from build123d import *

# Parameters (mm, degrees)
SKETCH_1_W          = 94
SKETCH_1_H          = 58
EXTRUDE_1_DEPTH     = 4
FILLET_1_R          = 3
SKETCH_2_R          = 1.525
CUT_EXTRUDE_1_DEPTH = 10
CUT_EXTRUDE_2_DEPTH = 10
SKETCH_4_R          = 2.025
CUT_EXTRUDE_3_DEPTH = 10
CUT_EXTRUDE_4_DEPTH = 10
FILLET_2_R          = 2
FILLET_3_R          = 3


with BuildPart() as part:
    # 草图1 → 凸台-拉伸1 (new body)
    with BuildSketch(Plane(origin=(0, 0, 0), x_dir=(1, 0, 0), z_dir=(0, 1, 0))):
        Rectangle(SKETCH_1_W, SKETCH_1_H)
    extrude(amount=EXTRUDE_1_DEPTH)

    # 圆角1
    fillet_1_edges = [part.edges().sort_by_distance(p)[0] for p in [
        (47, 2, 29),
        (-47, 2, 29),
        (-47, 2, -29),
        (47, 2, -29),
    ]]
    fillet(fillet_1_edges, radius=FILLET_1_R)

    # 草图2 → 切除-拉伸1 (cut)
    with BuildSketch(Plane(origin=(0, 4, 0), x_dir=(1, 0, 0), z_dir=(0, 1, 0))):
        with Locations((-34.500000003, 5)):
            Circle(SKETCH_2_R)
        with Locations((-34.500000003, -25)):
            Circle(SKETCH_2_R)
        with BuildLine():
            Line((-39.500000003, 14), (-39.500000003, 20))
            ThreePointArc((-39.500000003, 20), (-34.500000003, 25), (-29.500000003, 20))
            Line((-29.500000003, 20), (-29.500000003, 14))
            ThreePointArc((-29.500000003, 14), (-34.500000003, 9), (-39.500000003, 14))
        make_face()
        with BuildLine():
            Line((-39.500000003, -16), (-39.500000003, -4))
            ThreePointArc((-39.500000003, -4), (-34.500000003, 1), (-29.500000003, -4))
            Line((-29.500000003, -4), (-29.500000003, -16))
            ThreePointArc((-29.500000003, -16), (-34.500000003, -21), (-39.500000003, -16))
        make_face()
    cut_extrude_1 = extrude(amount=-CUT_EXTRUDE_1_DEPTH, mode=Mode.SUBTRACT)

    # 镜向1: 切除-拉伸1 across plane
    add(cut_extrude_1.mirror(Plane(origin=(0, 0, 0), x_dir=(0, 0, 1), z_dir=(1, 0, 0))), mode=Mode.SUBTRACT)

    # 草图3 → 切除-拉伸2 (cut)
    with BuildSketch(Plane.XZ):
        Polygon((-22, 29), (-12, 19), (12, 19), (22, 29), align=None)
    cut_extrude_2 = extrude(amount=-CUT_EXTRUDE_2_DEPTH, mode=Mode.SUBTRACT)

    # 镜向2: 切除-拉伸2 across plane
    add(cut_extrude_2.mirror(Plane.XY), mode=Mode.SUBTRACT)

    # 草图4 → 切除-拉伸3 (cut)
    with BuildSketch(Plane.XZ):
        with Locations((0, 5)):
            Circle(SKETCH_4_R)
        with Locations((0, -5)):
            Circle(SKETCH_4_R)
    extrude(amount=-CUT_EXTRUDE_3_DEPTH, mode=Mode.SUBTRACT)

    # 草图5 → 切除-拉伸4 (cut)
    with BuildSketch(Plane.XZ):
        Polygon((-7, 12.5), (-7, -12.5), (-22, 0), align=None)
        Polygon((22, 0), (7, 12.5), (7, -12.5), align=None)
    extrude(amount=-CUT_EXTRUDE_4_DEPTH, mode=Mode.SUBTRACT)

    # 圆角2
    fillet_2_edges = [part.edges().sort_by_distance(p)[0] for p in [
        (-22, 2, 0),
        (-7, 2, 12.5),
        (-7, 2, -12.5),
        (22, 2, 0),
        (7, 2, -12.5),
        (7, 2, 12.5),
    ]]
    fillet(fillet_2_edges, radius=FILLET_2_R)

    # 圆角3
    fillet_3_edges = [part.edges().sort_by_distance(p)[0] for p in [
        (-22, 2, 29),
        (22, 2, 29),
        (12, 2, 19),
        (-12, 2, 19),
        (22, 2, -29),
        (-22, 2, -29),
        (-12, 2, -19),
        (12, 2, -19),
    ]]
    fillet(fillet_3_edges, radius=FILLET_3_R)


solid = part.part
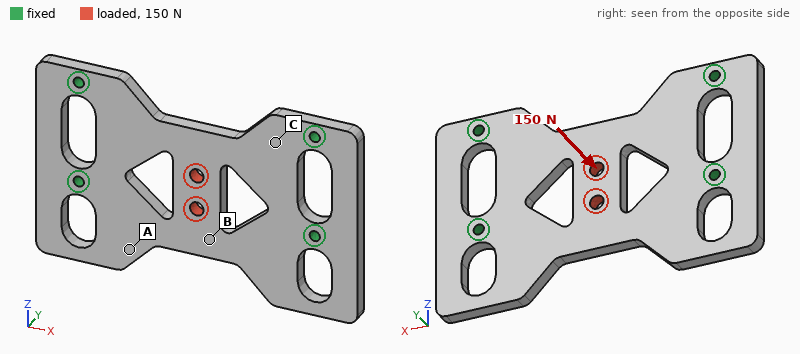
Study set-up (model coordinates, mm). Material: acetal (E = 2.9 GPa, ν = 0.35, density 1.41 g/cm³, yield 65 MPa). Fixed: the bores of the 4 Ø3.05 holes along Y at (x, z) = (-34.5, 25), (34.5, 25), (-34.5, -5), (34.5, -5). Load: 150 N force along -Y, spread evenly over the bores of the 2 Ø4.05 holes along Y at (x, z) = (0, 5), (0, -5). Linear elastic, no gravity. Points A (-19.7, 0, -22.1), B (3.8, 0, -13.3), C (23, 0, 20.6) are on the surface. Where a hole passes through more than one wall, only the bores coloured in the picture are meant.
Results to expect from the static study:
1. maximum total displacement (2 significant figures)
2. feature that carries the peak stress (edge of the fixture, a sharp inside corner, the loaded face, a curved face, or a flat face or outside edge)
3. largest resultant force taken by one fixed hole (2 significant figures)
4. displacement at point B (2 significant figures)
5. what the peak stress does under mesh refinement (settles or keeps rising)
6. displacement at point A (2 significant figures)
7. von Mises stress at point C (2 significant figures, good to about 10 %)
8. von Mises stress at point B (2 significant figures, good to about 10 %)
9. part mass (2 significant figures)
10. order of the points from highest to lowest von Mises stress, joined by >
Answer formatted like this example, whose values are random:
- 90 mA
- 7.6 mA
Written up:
- 0.88 mm
- edge of the fixture
- 58 N
- 0.78 mm
- keeps rising
- 0.39 mm
- 6.0 MPa
- 16 MPa
- 21 g
- B > C > A
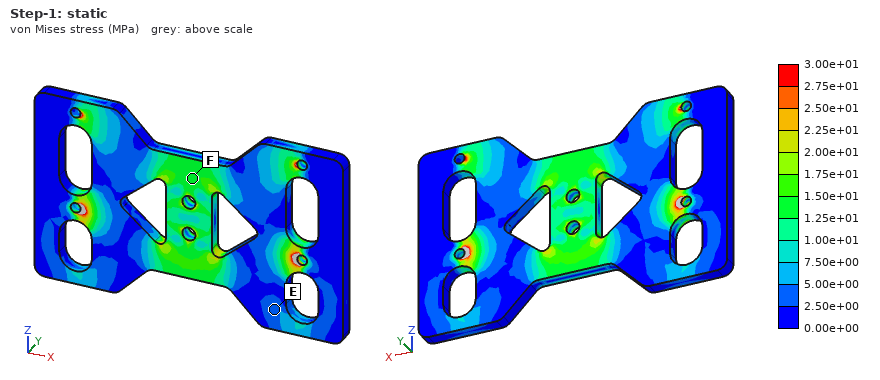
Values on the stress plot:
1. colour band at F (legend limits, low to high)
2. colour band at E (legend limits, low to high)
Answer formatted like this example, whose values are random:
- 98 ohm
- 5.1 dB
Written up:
- 1.25e+01 to 1.50e+01 MPa
- 2.50e+00 to 5.00e+00 MPa
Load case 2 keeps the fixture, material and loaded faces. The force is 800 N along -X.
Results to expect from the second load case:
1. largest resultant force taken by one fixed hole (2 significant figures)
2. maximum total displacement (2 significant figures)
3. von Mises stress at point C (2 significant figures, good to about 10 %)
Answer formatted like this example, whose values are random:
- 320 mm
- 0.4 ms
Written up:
- 230 N
- 0.18 mm
- 5.2 MPa
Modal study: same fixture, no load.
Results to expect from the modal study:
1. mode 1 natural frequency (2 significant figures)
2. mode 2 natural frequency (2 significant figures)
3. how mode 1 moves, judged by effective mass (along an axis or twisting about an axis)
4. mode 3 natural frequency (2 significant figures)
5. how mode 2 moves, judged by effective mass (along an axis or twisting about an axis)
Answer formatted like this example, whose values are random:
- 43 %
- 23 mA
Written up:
- 930 Hz
- 1200 Hz
- along Y
- 1400 Hz
- twisting about X
